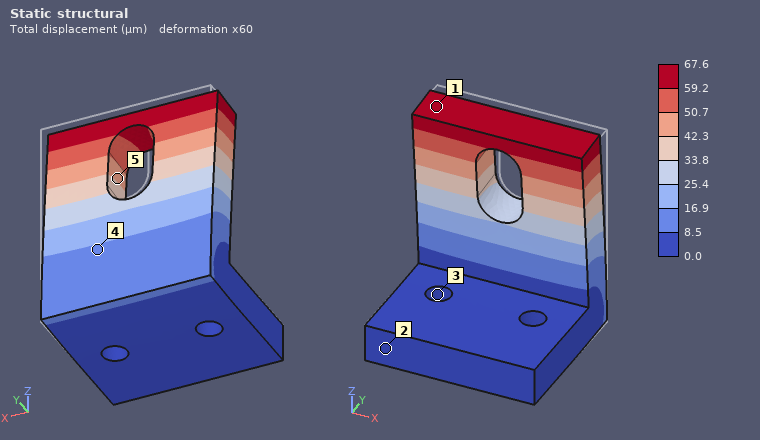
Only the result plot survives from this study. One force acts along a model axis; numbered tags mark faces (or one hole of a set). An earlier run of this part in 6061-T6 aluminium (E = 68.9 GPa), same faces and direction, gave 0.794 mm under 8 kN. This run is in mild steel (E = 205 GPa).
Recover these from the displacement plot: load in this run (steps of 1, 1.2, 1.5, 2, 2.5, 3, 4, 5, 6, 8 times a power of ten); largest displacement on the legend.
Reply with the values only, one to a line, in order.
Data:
2 kN
67.6 µm
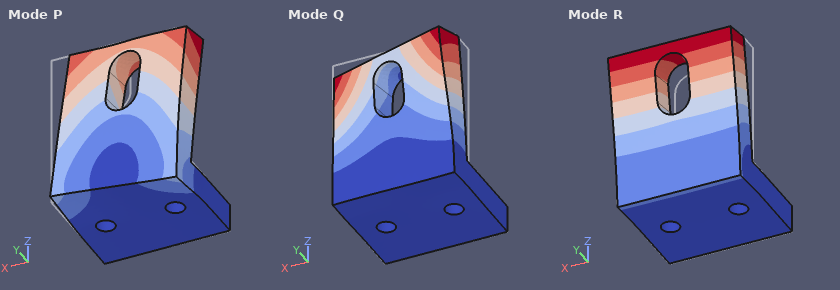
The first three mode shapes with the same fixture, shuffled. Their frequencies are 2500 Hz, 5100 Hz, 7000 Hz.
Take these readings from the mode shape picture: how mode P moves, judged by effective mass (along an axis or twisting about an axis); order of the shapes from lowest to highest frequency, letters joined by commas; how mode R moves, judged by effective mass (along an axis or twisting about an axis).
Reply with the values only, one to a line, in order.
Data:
along X
R, P, Q
along Y
